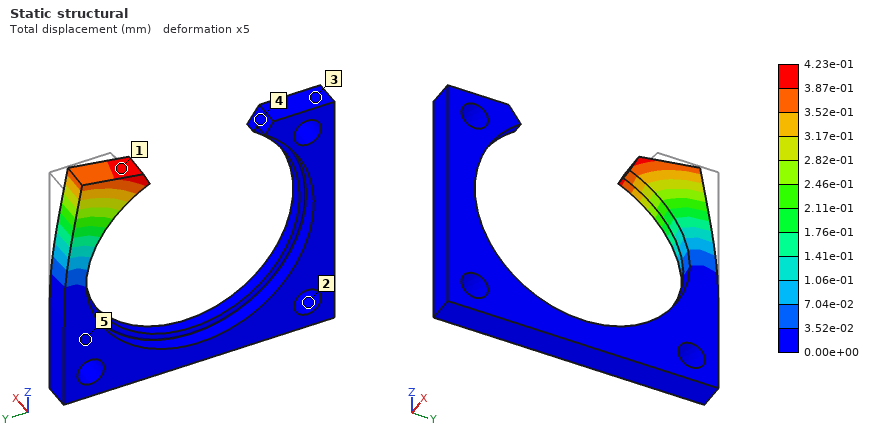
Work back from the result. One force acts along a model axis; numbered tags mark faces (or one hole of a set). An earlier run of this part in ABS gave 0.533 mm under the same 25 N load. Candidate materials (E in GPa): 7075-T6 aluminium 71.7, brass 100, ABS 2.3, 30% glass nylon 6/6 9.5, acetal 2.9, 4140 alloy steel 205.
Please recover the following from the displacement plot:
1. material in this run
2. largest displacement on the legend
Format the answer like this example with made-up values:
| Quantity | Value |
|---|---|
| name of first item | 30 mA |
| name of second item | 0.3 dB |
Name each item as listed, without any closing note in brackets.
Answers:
| Quantity | Value |
|---|---|
| material in this run | acetal |
| largest displacement on the legend | 4.23e-01 mm |
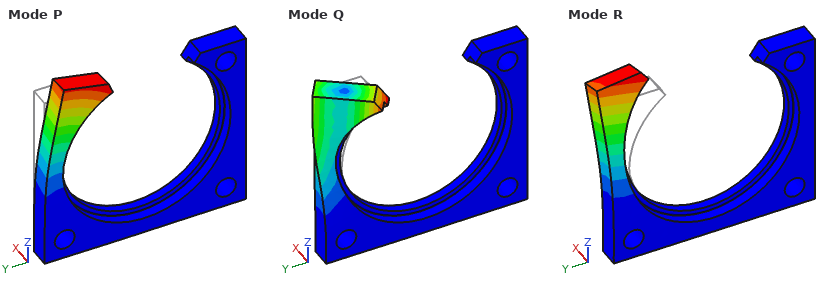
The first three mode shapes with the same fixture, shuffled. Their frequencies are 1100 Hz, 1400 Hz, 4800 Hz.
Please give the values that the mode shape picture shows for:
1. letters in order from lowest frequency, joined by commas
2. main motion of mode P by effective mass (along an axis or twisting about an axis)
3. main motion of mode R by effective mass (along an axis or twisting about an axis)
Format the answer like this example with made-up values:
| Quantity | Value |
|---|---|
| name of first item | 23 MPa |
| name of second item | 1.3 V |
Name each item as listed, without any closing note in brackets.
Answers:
| Quantity | Value |
|---|---|
| letters in order from lowest frequency, joined by commas | R, P, Q |
| main motion of mode P by effective mass | along Y |
| main motion of mode R by effective mass | along X |
